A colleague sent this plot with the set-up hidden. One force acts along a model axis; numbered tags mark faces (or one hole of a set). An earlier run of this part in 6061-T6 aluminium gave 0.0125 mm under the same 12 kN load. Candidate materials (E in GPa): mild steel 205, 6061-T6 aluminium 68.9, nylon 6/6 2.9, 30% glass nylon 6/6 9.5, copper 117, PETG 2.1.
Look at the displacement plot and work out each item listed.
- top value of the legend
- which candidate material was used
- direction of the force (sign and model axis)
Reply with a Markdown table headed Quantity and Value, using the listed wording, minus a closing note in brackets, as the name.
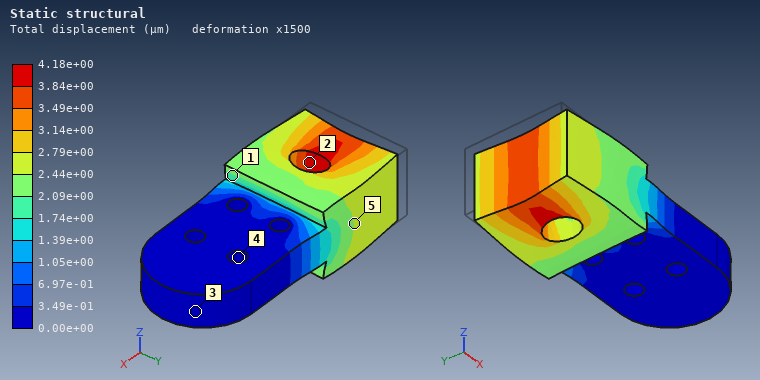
| Quantity | Value |
|---|---|
| top value of the legend | 4.18e+00 µm |
| which candidate material was used | mild steel |
| direction of the force | +X |
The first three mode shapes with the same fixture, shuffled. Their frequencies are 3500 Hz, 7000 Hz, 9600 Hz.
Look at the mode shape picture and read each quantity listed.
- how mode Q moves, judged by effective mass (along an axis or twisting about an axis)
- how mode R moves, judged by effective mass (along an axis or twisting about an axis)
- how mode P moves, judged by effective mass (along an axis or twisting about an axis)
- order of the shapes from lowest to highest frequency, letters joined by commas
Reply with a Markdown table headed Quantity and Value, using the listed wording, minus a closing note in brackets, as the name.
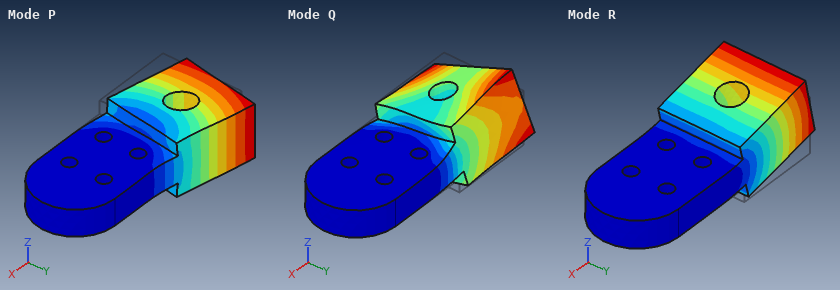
| Quantity | Value |
|---|---|
| how mode Q moves, judged by effective mass | twisting about X |
| how mode R moves, judged by effective mass | along Z |
| how mode P moves, judged by effective mass | along Y |
| order of the shapes from lowest to highest frequency, letters joined by commas | R, P, Q |
